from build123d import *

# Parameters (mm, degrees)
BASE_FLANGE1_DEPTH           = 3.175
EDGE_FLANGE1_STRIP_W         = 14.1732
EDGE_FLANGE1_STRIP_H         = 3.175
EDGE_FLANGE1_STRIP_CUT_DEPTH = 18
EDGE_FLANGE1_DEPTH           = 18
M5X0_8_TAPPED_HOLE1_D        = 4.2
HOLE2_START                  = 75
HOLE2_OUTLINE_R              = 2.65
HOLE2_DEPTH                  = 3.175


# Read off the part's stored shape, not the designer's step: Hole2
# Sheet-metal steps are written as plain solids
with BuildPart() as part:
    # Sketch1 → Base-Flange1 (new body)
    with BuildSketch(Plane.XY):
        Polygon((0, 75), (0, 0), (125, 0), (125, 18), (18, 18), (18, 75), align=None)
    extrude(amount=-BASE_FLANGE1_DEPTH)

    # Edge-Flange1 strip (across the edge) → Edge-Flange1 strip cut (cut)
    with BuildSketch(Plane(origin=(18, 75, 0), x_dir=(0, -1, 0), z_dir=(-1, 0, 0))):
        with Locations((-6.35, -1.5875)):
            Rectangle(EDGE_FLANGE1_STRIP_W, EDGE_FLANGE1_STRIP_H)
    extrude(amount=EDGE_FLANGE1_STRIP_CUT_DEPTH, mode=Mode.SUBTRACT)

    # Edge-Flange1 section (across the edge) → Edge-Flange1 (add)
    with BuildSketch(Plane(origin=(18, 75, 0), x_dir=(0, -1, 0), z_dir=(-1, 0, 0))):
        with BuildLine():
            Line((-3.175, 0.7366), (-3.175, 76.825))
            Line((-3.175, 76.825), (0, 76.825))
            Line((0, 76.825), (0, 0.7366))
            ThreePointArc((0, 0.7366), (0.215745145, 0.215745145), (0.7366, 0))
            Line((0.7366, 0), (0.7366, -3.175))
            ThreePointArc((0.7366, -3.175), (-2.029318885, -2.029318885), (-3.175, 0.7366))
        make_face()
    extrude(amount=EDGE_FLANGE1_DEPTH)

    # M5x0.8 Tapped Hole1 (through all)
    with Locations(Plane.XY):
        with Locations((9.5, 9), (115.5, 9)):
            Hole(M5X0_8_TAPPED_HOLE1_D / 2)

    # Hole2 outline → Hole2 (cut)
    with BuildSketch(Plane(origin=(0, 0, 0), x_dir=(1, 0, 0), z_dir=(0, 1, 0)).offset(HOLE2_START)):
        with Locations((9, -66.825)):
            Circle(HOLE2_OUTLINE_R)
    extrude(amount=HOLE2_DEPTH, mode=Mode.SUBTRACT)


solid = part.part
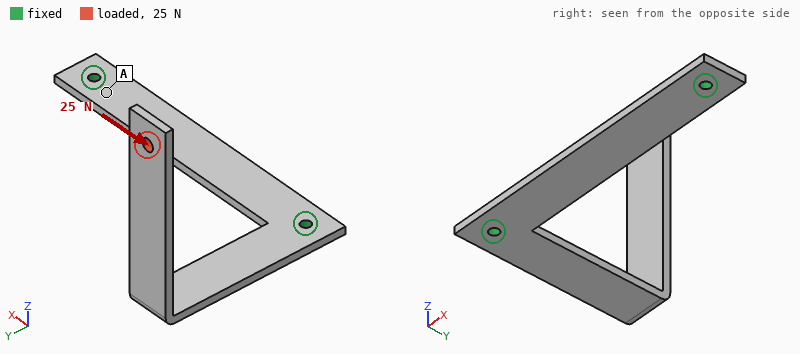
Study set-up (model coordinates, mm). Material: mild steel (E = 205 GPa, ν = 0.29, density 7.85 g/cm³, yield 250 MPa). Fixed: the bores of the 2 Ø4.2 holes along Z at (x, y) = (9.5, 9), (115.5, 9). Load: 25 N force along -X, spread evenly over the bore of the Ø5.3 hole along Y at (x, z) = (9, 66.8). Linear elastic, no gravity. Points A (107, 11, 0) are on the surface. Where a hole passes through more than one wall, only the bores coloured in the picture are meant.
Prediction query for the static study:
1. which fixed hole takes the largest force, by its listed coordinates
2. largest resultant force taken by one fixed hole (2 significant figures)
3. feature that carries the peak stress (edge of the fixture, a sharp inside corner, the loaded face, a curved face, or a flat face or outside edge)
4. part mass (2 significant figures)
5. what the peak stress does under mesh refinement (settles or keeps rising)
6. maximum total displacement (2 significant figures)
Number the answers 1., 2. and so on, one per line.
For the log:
1. (9.5, 9)
2. 20 N
3. edge of the fixture
4. 120 g
5. keeps rising
6. 0.64 mm
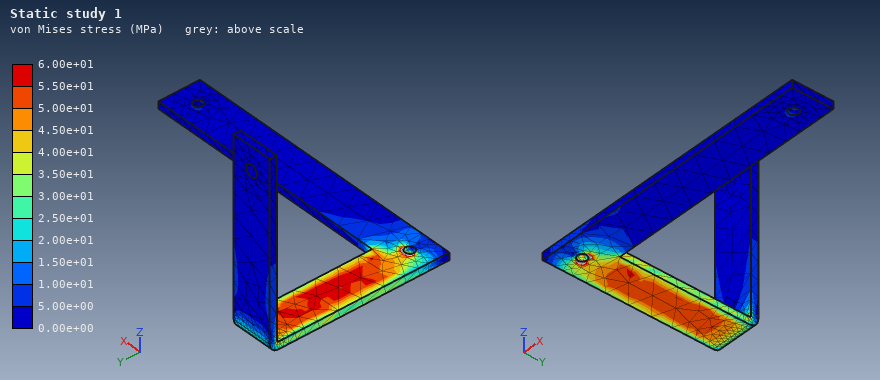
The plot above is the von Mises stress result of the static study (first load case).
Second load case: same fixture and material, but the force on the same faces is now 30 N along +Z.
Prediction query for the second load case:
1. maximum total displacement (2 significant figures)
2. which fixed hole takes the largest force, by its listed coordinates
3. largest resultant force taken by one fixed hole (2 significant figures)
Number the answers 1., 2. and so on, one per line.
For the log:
1. 0.60 mm
2. (9.5, 9)
3. 31 N
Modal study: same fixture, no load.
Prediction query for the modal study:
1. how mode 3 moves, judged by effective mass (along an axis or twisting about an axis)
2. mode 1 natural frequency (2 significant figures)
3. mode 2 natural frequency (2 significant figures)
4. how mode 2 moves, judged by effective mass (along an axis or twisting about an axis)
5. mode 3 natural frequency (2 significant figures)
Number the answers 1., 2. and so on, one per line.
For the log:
1. along Z
2. 170 Hz
3. 270 Hz
4. along X
5. 470 Hz
